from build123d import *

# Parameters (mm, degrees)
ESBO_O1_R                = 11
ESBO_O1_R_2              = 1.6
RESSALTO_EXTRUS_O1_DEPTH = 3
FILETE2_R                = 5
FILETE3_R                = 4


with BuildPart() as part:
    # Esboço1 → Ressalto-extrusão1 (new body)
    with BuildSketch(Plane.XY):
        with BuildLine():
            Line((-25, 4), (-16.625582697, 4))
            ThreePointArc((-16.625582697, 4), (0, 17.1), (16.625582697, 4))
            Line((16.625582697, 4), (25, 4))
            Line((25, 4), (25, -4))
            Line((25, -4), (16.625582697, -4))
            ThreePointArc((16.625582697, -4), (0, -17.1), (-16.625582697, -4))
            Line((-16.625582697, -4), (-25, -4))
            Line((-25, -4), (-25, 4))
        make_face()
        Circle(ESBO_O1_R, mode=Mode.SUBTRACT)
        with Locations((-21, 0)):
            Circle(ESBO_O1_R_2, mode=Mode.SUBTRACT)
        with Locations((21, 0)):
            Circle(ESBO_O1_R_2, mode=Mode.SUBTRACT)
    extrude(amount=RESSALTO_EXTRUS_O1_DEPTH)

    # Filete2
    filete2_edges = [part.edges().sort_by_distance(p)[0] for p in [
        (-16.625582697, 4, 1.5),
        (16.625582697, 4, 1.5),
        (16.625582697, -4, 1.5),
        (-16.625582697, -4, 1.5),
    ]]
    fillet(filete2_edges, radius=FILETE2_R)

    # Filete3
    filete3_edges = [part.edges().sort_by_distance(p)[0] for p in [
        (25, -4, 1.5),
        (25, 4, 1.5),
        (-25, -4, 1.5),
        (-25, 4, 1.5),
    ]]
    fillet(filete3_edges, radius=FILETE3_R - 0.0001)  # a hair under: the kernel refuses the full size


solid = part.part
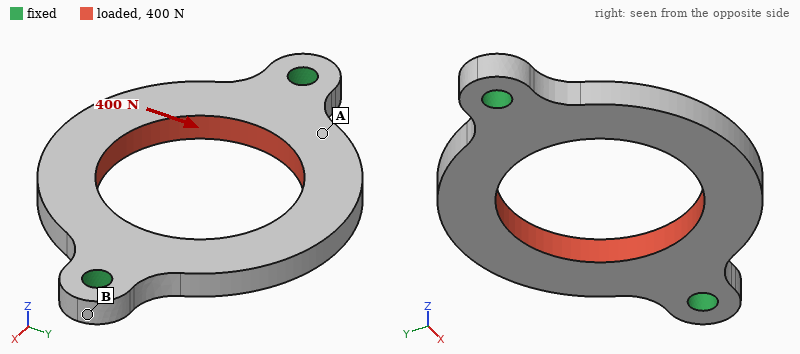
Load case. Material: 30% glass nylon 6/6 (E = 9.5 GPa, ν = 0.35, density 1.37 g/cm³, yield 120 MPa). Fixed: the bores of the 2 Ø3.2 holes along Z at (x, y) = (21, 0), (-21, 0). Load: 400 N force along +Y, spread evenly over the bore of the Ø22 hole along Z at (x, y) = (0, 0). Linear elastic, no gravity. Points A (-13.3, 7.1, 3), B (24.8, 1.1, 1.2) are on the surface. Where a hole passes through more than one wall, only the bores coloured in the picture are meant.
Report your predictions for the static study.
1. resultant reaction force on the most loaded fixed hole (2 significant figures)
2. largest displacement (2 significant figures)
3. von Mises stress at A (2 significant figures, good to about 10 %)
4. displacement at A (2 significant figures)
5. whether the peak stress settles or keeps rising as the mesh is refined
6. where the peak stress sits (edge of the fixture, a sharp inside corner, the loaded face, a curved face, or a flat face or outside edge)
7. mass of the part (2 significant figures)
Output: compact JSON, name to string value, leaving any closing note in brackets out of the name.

{"resultant reaction force on the most loaded fixed hole": "200 N", "largest displacement": "27 µm", "von Mises stress at A": "8.7 MPa", "displacement at A": "23 µm", "whether the peak stress settles or keeps rising as the mesh is refined": "keeps rising", "where the peak stress sits": "edge of the fixture", "mass of the part": "2.7 g"}
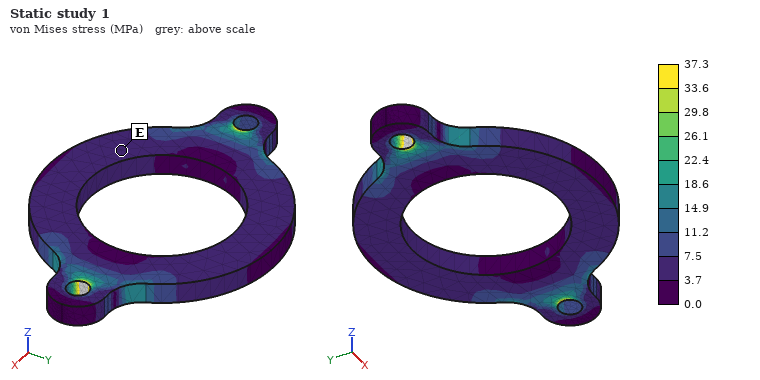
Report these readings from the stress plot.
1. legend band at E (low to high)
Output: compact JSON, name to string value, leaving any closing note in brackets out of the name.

{"legend band at E": "3.7 to 7.5 MPa"}
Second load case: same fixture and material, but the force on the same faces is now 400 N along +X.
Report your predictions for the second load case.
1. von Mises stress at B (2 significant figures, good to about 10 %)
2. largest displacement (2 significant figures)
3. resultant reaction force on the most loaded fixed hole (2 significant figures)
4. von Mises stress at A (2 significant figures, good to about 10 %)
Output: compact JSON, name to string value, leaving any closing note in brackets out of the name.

{"von Mises stress at B": "2.1 MPa", "largest displacement": "22 µm", "resultant reaction force on the most loaded fixed hole": "200 N", "von Mises stress at A": "6.7 MPa"}
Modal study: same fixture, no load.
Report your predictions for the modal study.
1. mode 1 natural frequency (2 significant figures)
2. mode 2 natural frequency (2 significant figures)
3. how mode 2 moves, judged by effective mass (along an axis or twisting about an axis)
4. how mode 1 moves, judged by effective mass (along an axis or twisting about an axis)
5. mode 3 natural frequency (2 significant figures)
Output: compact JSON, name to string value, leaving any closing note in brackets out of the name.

{"mode 1 natural frequency": "2500 Hz", "mode 2 natural frequency": "3000 Hz", "how mode 2 moves, judged by effective mass": "along Z", "how mode 1 moves, judged by effective mass": "twisting about X", "mode 3 natural frequency": "7400 Hz"}
